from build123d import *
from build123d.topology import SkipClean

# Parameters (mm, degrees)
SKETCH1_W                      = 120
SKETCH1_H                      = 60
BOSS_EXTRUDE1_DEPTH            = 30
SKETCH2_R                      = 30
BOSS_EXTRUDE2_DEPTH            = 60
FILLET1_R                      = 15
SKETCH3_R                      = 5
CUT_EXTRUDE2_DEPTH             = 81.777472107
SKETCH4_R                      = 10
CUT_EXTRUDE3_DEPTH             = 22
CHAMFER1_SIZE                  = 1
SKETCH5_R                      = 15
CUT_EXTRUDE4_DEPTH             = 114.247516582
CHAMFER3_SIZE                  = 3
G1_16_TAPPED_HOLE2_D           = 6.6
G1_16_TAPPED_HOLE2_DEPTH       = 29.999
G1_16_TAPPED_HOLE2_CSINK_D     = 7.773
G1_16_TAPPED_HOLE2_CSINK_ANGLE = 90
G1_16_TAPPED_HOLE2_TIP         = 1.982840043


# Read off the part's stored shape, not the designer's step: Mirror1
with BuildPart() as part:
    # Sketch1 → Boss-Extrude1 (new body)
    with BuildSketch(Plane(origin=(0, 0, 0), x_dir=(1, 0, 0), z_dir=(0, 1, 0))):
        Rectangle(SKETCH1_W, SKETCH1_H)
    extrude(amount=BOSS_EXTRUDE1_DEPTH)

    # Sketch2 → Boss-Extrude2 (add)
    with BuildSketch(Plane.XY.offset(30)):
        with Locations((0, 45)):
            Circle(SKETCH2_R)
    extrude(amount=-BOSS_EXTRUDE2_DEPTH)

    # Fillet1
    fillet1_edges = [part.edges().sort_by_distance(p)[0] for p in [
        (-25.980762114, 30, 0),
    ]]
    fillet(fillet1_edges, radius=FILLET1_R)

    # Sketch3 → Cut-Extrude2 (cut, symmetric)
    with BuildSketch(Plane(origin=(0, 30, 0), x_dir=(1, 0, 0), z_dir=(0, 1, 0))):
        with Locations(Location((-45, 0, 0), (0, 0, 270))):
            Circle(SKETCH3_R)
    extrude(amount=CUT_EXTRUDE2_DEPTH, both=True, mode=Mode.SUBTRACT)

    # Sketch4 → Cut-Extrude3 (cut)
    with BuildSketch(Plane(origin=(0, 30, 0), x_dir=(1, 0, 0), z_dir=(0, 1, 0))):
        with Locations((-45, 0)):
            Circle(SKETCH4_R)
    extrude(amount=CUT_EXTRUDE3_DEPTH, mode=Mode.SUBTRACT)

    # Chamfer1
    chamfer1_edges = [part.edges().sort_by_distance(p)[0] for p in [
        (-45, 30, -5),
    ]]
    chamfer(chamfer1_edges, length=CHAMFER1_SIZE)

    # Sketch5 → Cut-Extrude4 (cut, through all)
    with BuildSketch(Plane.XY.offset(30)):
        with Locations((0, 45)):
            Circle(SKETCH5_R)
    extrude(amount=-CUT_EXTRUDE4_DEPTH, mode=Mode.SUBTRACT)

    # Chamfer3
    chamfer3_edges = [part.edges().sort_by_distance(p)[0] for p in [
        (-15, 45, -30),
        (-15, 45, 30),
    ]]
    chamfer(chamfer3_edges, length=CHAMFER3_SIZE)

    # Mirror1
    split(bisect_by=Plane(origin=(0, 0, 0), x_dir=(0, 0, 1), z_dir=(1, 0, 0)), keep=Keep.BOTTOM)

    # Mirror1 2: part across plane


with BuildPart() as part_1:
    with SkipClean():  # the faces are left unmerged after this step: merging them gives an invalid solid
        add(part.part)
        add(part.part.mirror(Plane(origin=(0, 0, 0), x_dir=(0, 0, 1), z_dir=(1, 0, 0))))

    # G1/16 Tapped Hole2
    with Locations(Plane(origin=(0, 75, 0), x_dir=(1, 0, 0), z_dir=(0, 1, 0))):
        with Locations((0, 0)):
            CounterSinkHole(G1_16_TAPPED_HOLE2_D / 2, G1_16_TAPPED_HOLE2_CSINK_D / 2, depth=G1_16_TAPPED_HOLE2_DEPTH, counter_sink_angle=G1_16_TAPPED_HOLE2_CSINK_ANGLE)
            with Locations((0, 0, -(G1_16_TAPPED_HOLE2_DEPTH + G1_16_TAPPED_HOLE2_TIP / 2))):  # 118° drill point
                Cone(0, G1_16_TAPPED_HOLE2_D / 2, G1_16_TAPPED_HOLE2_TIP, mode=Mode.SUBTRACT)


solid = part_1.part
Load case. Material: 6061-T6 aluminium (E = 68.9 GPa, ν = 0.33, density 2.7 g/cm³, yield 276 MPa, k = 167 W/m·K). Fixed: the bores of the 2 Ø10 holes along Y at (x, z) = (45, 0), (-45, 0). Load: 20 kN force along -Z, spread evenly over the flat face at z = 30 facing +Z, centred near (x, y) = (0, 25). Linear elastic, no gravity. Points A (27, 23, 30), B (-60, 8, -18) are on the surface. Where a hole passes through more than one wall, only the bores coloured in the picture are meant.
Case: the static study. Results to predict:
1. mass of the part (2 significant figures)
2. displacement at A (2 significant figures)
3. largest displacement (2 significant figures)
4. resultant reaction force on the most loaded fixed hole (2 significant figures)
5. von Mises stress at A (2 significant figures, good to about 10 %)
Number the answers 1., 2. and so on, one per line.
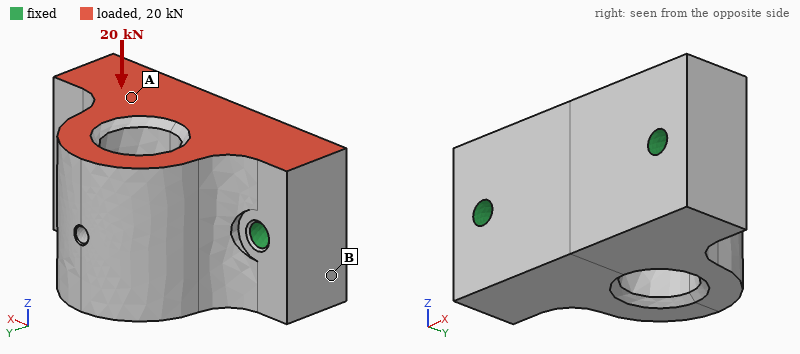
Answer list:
1. 840 g
2. 11 µm
3. 31 µm
4. 10 kN
5. 9.8 MPa
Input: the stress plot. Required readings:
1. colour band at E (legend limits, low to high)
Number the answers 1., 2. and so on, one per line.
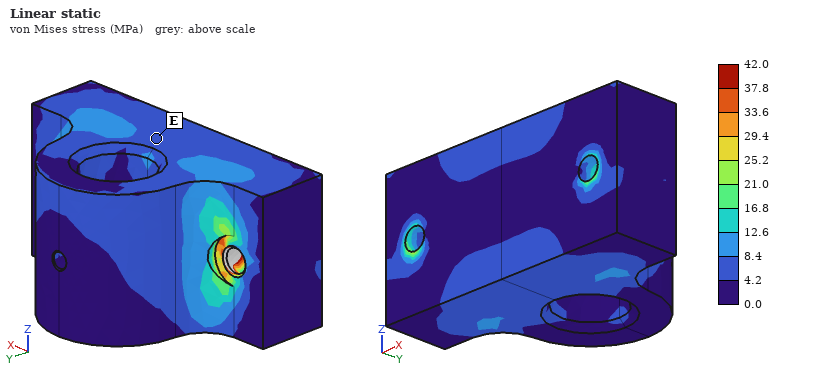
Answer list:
1. 4.2 to 8.4 MPa
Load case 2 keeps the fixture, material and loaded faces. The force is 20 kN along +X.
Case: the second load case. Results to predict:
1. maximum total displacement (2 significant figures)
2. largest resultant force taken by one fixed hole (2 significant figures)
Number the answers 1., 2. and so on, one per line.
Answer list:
1. 20 µm
2. 12 kN
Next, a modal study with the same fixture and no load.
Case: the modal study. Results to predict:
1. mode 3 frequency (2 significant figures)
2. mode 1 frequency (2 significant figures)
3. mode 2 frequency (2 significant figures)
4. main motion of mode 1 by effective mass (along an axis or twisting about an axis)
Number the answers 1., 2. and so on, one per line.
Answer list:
1. 9200 Hz
2. 5000 Hz
3. 9000 Hz
4. along Z
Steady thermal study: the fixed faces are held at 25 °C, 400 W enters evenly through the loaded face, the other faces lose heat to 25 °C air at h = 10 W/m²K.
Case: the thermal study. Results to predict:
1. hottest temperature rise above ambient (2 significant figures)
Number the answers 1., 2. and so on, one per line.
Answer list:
1. 31 K
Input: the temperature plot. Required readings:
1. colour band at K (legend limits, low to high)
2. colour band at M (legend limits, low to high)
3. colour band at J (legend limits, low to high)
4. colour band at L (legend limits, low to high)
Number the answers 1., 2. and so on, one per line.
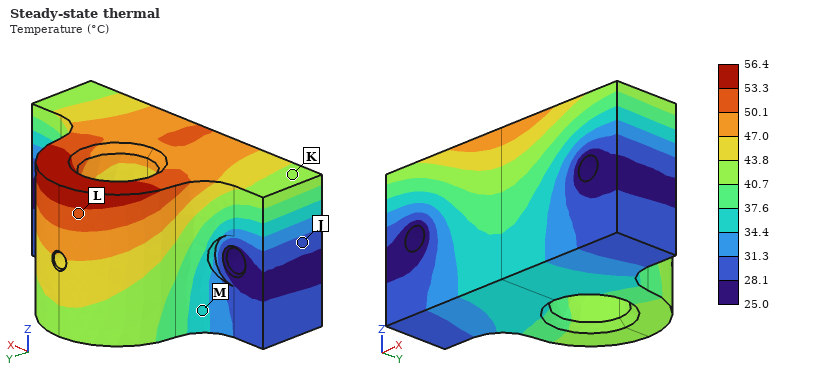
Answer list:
1. 40.7 to 43.8 °C
2. 34.4 to 37.6 °C
3. 28.1 to 31.3 °C
4. 50.1 to 53.3 °C
